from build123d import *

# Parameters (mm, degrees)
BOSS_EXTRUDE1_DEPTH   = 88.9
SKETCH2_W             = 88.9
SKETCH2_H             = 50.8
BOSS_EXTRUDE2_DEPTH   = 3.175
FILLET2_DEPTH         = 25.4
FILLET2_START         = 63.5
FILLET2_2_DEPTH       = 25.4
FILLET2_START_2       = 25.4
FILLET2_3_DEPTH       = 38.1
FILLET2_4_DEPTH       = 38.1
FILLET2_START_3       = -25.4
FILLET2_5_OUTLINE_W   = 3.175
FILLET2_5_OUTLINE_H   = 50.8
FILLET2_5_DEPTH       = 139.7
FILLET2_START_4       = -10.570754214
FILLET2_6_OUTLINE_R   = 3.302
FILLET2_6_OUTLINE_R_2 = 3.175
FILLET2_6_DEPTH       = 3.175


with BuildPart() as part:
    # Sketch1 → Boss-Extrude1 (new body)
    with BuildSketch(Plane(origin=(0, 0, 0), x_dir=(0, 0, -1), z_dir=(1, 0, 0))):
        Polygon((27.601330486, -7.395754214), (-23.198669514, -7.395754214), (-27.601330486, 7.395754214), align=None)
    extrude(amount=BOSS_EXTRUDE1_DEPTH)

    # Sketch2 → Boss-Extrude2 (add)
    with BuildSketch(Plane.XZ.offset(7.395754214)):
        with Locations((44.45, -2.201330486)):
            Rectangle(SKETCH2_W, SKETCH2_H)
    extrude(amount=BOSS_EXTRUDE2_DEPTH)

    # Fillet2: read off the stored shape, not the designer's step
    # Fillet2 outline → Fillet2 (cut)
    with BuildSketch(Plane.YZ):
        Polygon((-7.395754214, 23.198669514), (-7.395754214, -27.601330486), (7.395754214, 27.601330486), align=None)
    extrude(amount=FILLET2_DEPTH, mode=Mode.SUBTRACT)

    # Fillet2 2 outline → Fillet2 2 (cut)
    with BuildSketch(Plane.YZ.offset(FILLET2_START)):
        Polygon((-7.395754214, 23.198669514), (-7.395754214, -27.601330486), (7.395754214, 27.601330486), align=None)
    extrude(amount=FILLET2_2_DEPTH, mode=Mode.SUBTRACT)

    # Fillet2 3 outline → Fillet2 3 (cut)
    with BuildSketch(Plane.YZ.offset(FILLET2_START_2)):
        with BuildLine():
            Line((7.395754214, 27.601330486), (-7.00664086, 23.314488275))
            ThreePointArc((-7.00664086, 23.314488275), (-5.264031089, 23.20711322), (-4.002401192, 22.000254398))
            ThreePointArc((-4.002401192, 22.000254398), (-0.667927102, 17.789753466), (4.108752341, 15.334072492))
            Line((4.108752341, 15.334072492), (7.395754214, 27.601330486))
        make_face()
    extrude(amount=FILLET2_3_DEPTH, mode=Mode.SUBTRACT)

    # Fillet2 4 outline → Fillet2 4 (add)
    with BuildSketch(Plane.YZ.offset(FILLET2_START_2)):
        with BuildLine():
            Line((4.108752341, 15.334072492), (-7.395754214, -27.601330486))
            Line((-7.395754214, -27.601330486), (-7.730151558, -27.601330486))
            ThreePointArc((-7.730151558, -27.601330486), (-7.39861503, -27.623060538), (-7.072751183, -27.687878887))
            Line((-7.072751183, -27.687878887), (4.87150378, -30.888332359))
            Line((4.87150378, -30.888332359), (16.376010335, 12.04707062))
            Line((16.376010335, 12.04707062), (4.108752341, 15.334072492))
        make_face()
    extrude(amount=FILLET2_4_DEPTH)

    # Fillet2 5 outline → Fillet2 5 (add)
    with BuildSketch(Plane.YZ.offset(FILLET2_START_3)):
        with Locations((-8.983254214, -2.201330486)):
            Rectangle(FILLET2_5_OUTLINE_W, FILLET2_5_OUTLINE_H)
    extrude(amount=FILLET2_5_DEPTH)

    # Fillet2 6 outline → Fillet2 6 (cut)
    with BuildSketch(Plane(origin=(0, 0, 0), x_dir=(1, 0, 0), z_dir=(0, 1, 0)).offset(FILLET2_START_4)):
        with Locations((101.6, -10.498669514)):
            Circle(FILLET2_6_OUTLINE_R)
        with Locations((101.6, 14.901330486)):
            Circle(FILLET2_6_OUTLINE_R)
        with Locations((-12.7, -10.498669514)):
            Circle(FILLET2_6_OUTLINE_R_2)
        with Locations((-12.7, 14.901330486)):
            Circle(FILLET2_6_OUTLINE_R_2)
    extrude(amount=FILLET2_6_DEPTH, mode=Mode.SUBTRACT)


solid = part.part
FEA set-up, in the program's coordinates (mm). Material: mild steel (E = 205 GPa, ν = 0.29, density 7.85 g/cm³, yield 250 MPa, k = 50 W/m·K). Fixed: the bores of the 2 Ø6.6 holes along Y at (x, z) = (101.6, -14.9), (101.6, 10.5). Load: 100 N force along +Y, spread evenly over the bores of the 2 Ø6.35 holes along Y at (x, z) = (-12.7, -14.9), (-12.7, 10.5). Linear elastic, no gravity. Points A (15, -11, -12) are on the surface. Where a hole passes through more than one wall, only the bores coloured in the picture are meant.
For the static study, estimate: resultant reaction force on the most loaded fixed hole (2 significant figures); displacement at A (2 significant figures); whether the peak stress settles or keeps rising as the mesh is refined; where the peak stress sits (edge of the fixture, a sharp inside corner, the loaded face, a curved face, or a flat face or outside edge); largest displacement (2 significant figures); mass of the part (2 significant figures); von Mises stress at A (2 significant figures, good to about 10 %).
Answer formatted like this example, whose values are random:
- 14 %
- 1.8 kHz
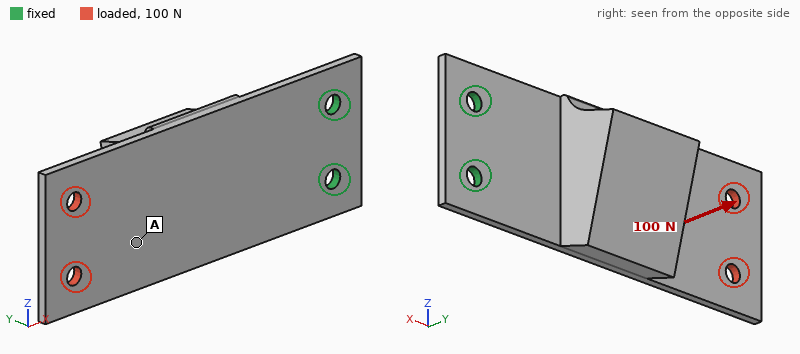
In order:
- 50 N
- 0.84 mm
- keeps rising
- edge of the fixture
- 1.4 mm
- 430 g
- 29 MPa
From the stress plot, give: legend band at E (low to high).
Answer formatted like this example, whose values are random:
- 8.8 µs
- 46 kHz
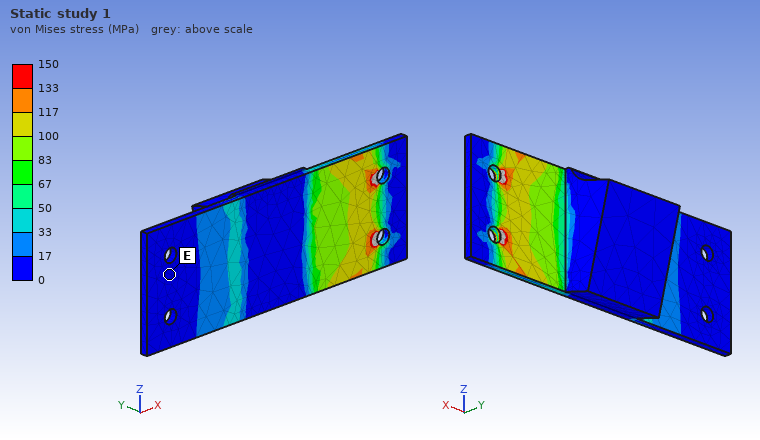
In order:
- 0 to 17 MPa
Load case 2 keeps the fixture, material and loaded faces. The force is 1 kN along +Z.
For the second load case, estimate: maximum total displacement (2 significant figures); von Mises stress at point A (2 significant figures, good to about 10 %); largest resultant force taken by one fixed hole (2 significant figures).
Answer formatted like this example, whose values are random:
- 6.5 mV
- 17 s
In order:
- 98 µm
- 14 MPa
- 3.9 kN
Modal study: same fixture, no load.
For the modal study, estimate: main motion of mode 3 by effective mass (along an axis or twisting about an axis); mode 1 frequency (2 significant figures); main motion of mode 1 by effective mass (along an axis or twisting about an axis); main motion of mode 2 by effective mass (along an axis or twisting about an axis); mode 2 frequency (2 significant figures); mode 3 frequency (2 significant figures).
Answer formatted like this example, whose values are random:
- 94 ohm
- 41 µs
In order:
- along Y
- 140 Hz
- along Y
- along Z
- 730 Hz
- 1000 Hz
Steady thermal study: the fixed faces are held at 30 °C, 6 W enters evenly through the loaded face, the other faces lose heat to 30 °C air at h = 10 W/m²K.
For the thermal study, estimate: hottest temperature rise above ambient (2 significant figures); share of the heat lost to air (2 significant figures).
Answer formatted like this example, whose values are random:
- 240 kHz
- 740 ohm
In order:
- 44 K
- 54 %
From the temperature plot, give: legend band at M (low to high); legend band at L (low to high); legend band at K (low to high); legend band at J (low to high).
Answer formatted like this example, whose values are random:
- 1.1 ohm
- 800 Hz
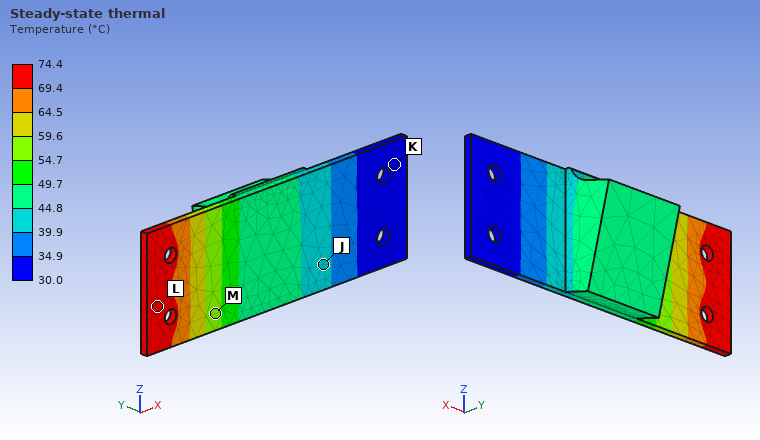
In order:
- 54.7 to 59.6 °C
- 69.4 to 74.4 °C
- 30.0 to 34.9 °C
- 39.9 to 44.8 °C
